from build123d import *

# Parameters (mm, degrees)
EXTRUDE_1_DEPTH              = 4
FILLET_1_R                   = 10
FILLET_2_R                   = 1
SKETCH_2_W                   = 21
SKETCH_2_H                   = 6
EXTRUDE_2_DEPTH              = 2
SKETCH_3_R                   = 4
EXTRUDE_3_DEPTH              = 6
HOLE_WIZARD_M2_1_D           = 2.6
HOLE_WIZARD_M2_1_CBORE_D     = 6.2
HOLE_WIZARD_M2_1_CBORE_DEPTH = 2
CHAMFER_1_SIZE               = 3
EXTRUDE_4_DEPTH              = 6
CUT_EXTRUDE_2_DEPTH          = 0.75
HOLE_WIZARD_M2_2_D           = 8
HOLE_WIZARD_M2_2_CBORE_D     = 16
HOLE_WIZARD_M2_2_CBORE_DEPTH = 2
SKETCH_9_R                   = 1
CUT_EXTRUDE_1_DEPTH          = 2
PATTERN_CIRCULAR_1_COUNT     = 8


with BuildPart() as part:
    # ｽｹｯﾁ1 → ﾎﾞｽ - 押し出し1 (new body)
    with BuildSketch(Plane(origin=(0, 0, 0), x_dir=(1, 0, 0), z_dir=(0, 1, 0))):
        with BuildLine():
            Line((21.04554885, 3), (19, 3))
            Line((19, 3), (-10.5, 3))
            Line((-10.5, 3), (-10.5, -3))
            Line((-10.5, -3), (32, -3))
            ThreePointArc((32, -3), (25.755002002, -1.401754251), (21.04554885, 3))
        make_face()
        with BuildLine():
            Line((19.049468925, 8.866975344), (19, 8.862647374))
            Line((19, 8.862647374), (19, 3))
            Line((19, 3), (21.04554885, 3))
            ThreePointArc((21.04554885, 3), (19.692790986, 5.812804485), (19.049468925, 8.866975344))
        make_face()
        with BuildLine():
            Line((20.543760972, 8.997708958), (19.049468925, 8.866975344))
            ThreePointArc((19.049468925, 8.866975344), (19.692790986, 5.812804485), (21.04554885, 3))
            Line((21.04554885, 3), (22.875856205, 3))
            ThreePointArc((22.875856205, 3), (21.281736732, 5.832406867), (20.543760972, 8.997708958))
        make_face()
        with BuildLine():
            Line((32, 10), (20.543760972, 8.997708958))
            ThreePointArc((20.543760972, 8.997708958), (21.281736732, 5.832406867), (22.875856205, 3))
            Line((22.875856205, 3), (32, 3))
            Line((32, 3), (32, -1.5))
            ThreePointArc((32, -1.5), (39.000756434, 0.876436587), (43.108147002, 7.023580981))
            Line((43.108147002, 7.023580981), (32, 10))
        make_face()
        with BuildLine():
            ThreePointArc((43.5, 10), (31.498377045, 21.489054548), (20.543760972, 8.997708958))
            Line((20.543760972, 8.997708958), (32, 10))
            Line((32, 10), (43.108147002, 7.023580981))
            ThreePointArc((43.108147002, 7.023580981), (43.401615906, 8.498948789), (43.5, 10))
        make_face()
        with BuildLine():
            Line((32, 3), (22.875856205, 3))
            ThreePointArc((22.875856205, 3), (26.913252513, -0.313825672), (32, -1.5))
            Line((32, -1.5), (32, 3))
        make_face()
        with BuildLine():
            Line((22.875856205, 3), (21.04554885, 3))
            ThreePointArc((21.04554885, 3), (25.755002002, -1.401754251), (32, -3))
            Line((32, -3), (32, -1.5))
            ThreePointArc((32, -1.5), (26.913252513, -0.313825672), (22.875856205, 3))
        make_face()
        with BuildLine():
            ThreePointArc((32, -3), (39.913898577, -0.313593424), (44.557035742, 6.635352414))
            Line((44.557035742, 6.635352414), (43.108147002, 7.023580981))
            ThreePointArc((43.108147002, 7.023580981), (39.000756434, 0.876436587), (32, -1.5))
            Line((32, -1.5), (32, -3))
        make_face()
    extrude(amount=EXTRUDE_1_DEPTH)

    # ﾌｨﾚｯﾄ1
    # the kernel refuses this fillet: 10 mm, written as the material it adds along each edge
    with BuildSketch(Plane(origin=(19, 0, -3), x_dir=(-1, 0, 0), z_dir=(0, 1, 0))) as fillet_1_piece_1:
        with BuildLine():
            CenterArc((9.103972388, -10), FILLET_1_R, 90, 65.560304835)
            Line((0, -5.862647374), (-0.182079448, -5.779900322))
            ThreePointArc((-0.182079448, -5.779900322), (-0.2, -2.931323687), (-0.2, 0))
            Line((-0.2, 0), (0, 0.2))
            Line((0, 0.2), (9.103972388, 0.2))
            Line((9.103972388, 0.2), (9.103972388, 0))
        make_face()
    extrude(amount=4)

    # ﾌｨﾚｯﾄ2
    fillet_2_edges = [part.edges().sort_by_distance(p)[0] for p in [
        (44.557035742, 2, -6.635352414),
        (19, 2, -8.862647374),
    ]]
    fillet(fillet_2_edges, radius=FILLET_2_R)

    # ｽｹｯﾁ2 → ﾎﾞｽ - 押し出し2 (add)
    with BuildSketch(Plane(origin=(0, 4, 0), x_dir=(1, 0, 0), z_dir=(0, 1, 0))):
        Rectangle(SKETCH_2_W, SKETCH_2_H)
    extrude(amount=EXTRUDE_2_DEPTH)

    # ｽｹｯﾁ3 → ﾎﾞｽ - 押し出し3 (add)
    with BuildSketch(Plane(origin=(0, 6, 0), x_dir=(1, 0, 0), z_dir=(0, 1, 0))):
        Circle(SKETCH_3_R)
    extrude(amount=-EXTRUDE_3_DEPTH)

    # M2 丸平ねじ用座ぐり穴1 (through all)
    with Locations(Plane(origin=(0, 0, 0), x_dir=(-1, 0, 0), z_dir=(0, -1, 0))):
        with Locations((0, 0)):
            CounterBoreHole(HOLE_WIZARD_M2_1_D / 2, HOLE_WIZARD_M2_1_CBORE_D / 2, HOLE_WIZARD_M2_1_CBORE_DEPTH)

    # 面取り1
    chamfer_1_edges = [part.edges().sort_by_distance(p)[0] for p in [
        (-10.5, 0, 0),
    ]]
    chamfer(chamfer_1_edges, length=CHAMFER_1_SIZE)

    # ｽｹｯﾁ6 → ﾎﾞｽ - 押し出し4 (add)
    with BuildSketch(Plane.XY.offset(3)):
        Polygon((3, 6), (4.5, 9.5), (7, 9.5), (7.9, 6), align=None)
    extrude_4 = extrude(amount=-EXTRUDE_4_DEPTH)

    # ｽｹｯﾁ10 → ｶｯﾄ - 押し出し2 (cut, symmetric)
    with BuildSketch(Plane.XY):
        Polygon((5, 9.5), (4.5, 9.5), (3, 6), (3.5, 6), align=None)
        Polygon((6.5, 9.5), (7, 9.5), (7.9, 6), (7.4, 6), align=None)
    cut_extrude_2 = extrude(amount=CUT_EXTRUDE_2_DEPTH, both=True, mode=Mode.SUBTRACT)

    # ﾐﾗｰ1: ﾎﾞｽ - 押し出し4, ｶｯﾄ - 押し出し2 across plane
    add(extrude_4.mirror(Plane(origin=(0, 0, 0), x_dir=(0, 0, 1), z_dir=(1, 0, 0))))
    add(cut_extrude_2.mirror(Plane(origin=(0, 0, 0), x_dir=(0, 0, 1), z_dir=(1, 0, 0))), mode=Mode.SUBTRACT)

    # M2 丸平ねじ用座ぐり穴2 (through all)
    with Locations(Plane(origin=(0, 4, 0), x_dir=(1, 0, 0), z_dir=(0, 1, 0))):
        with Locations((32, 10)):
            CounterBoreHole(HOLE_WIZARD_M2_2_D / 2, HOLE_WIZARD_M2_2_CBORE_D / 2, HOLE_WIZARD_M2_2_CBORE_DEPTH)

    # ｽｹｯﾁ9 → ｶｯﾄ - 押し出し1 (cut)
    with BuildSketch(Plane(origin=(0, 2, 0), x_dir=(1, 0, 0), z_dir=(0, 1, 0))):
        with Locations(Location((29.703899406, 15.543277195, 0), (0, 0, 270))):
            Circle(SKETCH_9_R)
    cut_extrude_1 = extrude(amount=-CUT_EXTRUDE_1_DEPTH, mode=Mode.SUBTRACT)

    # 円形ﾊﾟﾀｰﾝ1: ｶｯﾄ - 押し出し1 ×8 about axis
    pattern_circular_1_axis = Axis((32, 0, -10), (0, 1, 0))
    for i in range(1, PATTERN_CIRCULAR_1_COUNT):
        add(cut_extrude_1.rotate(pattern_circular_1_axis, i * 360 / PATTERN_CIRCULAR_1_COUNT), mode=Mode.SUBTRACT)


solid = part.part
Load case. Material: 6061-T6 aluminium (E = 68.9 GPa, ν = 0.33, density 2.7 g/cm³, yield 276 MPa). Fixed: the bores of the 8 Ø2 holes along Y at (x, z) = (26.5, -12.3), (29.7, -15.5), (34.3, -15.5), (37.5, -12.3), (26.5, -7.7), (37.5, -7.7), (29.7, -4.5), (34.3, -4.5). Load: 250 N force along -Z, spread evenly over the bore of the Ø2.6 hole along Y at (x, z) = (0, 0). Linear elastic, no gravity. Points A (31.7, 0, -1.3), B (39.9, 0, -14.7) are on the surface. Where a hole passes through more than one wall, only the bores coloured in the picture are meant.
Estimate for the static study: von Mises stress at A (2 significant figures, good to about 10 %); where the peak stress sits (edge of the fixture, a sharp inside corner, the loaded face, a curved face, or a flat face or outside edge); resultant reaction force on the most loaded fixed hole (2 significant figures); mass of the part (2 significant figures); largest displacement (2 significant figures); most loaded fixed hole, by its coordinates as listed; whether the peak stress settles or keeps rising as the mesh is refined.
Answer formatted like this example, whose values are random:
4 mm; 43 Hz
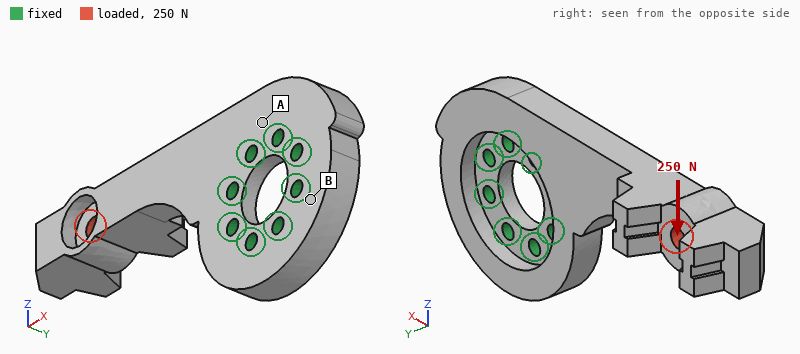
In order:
34 MPa; a sharp inside corner; 360 N; 6.9 g; 0.21 mm; (26.5, -12.3); keeps rising
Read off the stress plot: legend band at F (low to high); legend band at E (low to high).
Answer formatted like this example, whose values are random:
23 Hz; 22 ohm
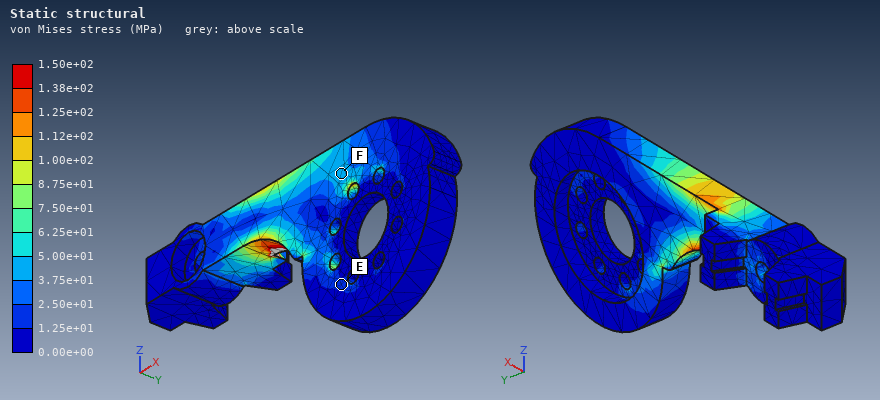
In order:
3.75e+01 to 5.00e+01 MPa; 1.25e+01 to 2.50e+01 MPa
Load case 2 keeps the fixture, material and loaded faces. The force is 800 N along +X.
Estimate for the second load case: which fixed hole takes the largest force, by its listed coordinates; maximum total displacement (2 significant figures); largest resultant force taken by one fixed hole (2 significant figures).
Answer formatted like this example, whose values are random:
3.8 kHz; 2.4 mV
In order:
(29.7, -4.5); 0.36 mm; 440 N
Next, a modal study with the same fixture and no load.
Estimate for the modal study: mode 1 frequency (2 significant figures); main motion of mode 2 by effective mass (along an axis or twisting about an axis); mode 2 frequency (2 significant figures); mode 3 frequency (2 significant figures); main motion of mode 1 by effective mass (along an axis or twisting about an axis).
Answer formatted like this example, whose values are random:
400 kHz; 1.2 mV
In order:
1900 Hz; along Z; 4500 Hz; 10 kHz; along Y
